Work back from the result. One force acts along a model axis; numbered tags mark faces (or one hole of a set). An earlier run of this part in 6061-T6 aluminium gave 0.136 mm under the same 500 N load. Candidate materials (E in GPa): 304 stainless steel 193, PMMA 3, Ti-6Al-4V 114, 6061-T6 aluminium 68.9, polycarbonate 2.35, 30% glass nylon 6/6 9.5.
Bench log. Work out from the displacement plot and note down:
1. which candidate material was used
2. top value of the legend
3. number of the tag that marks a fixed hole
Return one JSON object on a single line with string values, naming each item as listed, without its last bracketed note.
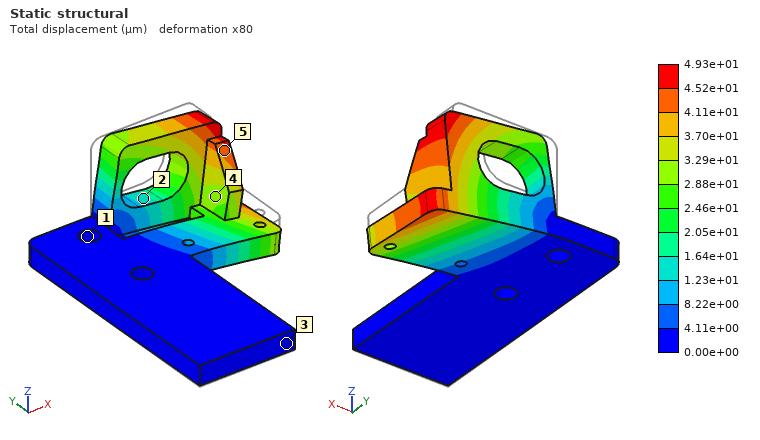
{"which candidate material was used": "304 stainless steel", "top value of the legend": "4.93e+01 µm", "number of the tag that marks a fixed hole": "1"}
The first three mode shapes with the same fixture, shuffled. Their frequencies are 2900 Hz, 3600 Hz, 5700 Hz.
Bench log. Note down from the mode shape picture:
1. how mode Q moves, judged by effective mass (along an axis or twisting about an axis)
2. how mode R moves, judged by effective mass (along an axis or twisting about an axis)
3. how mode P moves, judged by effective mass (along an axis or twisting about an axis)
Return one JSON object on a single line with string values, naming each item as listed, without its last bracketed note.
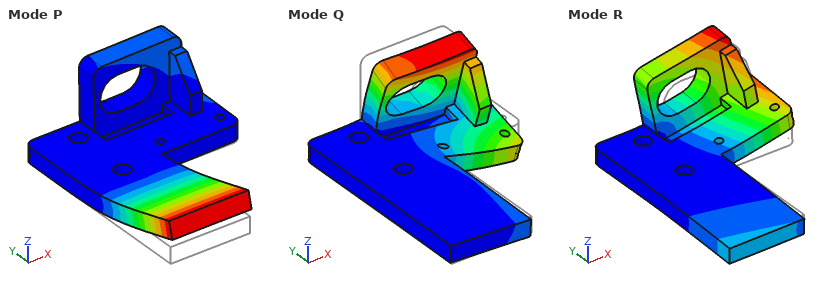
{"how mode Q moves, judged by effective mass": "along Y", "how mode R moves, judged by effective mass": "along Z", "how mode P moves, judged by effective mass": "along Z"}
